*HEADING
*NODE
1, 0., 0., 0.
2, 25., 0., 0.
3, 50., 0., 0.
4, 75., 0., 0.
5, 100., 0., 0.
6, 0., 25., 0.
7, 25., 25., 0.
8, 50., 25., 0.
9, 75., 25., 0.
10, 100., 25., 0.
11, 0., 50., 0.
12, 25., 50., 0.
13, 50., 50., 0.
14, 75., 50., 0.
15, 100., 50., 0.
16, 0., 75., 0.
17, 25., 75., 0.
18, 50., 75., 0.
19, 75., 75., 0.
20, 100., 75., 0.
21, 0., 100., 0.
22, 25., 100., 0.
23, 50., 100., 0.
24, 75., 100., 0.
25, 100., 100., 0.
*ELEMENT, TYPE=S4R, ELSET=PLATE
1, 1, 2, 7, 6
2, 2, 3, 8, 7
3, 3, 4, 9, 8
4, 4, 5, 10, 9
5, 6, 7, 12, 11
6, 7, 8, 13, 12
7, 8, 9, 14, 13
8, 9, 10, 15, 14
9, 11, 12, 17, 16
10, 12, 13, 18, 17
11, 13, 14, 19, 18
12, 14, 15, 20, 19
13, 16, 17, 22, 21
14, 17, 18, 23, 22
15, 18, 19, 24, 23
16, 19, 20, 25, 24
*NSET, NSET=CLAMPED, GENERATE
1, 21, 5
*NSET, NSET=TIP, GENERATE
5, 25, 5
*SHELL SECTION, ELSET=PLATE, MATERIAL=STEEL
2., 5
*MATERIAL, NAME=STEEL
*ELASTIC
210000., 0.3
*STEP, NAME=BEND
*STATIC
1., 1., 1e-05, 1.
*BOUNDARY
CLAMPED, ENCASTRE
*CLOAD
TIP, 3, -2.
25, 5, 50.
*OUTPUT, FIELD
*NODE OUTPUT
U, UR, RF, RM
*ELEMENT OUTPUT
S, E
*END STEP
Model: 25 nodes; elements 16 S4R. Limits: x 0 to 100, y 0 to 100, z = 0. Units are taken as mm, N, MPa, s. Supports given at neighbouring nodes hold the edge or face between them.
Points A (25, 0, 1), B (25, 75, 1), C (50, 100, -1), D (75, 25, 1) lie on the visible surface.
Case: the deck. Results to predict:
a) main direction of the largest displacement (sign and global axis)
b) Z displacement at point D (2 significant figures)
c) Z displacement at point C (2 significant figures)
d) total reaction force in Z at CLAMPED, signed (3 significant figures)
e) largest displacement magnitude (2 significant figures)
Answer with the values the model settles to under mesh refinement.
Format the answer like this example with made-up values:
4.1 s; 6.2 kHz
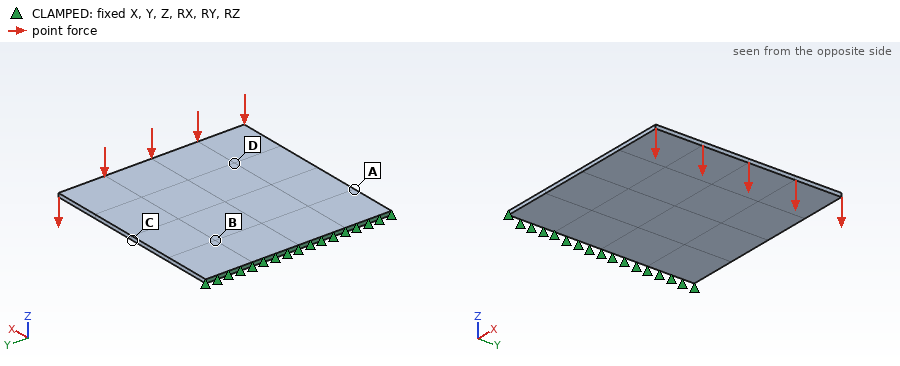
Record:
-Z; -0.15 mm; -0.067 mm; 10.0 N; 0.24 mm
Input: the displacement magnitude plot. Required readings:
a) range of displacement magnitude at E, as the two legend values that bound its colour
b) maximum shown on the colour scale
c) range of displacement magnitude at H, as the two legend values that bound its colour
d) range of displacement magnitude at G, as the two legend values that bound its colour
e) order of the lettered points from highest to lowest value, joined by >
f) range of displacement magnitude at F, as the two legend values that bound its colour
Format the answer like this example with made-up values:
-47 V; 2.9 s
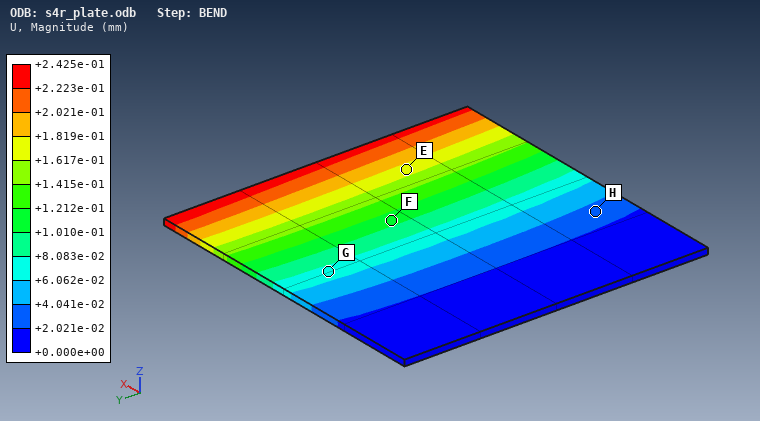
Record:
+1.617e-01 to +1.819e-01 mm; +2.425e-01 mm; +2.021e-02 to +4.041e-02 mm; +6.062e-02 to +8.083e-02 mm; E > F > G > H; +1.010e-01 to +1.212e-01 mm
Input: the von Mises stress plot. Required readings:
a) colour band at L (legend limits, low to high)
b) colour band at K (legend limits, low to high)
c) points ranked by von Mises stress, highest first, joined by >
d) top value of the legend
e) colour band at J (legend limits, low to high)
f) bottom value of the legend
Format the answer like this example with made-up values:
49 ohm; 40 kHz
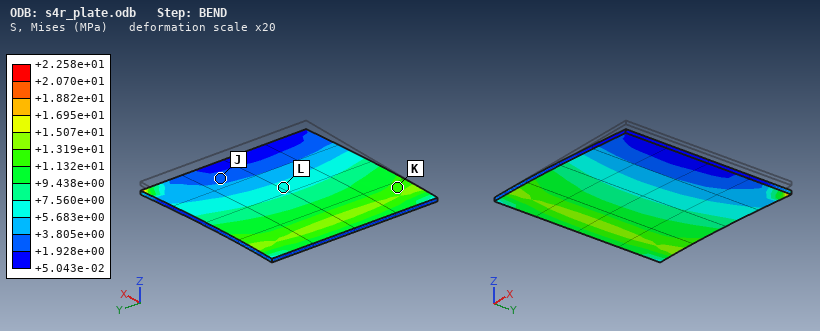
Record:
+5.683e+00 to +7.560e+00 MPa; +1.132e+01 to +1.319e+01 MPa; K > L > J; +2.258e+01 MPa; +1.928e+00 to +3.805e+00 MPa; +5.043e-02 MPa
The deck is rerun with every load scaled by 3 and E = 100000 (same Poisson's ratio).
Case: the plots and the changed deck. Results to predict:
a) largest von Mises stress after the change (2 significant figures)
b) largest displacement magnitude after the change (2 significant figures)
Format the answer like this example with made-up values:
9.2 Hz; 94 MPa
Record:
68 MPa; 1.5 mm
